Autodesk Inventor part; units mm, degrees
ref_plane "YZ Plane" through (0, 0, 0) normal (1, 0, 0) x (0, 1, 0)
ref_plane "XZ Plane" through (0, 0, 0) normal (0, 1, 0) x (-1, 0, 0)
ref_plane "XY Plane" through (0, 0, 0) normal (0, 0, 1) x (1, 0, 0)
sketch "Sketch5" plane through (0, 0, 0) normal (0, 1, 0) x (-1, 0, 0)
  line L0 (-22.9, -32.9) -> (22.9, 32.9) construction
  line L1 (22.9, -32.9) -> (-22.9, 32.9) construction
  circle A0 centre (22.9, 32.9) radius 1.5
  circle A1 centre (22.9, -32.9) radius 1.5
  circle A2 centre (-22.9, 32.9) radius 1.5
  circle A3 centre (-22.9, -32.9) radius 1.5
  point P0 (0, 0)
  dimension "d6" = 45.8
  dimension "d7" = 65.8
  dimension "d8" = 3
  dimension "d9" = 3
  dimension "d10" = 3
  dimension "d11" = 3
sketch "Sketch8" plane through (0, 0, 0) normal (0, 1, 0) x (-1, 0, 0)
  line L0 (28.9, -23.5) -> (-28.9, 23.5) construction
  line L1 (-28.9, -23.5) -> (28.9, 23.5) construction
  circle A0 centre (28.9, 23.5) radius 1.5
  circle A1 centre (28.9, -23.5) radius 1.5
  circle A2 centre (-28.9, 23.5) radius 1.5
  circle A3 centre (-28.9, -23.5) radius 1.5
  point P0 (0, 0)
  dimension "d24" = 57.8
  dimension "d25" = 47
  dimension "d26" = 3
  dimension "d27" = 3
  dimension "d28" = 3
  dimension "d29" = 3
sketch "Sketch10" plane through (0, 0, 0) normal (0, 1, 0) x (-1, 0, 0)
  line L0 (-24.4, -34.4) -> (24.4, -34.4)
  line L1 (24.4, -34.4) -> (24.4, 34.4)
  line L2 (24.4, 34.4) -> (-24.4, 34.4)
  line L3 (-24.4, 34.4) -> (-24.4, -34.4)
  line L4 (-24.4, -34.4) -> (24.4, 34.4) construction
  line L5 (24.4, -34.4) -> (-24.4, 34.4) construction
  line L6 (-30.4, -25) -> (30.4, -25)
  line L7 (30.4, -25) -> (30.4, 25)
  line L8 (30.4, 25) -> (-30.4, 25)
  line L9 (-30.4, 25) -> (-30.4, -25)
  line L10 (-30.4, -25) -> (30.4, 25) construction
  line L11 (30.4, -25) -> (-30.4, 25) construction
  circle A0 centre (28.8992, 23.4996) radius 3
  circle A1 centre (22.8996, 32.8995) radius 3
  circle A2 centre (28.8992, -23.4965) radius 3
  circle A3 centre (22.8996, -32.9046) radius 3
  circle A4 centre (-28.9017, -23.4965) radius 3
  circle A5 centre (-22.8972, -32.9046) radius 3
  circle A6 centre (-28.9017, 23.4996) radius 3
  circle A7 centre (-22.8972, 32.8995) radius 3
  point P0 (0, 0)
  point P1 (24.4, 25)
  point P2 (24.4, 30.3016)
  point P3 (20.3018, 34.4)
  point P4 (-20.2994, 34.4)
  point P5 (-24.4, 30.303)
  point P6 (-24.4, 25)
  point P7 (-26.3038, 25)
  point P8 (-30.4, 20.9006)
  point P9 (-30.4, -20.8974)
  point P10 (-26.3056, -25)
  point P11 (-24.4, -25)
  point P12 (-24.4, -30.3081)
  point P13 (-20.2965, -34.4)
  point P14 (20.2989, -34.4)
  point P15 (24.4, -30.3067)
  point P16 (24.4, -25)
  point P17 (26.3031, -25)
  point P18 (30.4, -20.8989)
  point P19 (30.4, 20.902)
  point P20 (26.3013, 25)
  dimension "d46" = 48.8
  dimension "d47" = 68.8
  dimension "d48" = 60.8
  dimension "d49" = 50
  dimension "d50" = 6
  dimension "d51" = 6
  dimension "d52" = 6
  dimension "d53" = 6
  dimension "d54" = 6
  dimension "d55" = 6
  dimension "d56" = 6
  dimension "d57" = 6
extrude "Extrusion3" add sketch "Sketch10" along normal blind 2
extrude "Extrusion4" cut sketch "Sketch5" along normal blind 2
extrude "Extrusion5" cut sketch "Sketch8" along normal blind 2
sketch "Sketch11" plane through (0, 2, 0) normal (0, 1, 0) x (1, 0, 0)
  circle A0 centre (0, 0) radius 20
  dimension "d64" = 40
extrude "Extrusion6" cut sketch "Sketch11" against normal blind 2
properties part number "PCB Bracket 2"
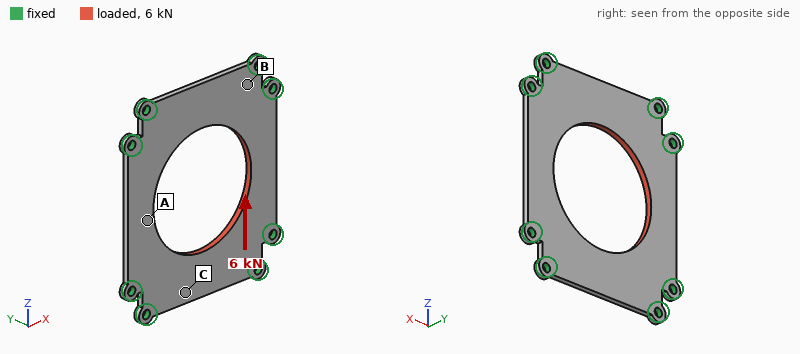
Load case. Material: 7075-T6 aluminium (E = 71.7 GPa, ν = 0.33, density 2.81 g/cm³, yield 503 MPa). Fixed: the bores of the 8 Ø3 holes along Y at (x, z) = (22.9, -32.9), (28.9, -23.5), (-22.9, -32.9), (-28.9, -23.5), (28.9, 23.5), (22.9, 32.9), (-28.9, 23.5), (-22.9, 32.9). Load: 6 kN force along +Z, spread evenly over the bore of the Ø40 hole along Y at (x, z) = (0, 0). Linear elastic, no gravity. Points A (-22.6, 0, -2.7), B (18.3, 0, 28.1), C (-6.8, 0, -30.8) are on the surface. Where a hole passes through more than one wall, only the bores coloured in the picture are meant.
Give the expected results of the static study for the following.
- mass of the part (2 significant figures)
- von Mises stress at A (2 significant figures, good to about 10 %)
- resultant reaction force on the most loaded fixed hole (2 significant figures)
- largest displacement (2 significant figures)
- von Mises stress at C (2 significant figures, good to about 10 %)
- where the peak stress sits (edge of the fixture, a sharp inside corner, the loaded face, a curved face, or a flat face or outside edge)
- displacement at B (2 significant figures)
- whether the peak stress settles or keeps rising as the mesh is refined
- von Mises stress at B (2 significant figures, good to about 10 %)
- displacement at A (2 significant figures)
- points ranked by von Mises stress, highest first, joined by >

15 g
43 MPa
1.1 kN
28 µm
21 MPa
edge of the fixture
8.1 µm
keeps rising
59 MPa
11 µm
B > A > C
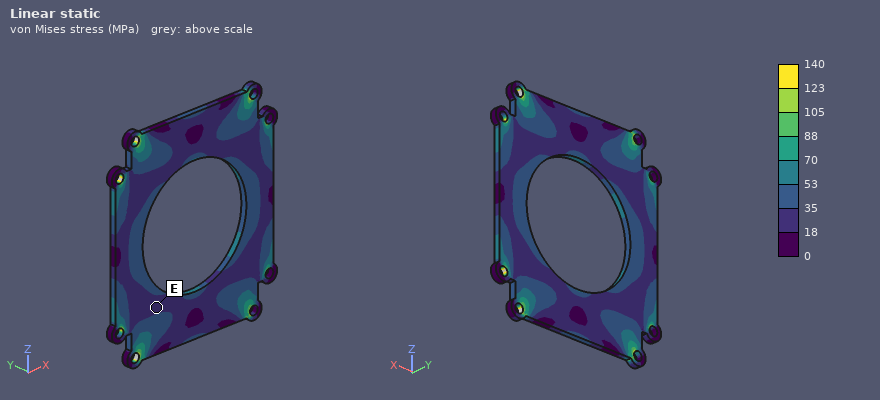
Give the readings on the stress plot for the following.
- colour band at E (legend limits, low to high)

18 to 35 MPa
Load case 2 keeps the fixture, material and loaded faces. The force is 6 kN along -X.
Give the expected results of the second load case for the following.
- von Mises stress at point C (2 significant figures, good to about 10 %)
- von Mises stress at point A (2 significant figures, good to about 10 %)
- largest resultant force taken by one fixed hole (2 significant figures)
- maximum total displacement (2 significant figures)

28 MPa
28 MPa
1.2 kN
38 µm
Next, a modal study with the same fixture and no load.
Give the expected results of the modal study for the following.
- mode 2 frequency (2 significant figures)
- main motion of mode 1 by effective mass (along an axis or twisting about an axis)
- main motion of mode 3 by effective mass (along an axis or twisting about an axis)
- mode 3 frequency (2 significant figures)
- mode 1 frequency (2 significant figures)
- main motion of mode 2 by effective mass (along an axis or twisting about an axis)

4500 Hz
along Y
twisting about Z
4800 Hz
3800 Hz
twisting about X
